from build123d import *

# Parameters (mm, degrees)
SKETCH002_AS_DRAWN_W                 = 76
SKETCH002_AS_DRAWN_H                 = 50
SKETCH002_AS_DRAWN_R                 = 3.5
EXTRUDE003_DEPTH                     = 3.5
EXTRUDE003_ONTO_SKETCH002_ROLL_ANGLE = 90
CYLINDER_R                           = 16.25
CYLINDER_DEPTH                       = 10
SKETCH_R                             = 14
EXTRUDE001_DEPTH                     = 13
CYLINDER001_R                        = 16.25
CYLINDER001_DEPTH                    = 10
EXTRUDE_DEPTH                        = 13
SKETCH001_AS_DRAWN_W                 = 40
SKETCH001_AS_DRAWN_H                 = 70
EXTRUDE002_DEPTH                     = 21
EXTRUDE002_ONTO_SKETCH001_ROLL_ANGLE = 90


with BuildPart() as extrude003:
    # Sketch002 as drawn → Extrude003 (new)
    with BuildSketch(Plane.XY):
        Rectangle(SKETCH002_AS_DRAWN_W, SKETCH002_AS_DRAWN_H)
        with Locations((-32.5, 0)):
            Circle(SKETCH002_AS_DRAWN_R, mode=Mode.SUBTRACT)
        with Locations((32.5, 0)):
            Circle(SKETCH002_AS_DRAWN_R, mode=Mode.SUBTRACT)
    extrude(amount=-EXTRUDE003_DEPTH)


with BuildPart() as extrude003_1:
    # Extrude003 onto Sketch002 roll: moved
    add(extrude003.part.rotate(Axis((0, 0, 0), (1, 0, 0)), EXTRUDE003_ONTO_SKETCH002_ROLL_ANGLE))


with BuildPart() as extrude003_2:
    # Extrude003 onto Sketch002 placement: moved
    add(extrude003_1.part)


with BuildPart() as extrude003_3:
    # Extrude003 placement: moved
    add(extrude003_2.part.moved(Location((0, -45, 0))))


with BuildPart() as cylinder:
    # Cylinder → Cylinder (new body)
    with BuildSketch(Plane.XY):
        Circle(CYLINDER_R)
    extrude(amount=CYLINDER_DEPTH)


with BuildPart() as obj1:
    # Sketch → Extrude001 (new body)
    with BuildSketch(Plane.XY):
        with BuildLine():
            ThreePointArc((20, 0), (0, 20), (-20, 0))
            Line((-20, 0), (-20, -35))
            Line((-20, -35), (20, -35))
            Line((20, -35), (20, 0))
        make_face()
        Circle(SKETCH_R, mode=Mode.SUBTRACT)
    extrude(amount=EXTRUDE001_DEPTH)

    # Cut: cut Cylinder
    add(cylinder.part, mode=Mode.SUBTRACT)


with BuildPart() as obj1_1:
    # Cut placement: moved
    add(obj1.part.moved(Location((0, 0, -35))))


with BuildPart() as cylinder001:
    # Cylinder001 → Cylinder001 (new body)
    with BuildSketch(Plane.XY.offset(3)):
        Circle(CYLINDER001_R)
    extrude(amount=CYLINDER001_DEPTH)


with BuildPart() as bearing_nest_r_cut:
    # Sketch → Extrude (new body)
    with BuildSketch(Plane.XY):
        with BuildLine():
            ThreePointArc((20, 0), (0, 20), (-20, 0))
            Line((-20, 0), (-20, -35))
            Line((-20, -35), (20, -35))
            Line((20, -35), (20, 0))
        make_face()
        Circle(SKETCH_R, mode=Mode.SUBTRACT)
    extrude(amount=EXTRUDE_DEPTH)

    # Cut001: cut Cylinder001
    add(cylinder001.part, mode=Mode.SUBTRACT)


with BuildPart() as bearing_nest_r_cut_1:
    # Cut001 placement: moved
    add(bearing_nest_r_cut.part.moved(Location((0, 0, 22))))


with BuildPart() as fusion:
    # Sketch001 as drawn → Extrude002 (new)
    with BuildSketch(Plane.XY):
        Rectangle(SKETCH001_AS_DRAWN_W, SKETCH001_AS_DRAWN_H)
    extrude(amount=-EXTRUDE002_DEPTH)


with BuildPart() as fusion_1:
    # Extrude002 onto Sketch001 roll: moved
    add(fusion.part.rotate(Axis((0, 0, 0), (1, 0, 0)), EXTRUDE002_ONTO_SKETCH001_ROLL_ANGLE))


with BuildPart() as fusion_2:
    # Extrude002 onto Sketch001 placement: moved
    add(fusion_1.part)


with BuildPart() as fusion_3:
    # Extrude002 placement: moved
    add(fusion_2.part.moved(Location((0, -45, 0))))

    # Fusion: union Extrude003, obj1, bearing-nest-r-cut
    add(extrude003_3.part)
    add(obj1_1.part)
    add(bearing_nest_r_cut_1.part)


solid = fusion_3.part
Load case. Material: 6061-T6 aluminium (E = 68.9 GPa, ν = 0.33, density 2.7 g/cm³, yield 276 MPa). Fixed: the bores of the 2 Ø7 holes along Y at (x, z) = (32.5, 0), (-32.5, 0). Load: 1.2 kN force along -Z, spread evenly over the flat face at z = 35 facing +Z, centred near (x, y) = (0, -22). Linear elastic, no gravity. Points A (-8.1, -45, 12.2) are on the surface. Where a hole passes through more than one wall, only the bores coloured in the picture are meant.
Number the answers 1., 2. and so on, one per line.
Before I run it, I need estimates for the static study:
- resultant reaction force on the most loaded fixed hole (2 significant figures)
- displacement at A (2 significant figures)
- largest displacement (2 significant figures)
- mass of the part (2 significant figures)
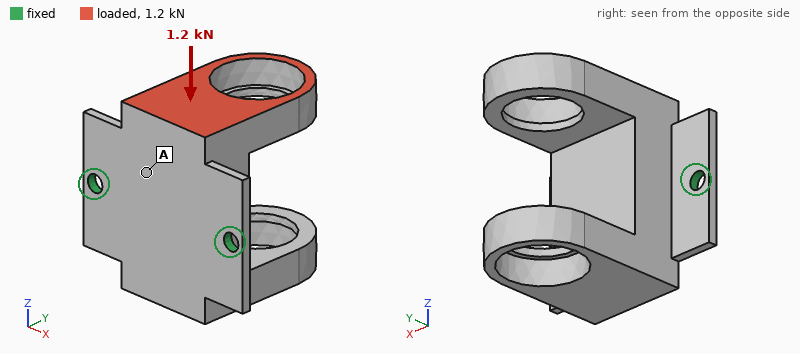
1. 600 N
2. 0.091 mm
3. 0.58 mm
4. 230 g
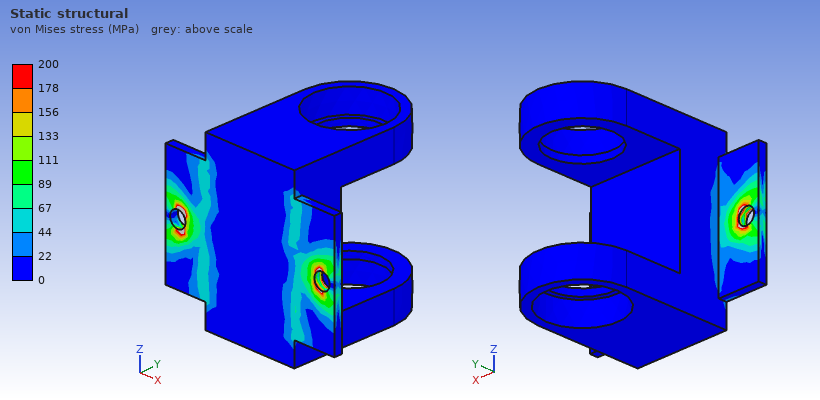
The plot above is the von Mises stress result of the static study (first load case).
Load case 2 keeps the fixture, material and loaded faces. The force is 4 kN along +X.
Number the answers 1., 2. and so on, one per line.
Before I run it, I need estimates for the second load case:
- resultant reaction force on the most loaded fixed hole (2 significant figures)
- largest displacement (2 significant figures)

1. 3.4 kN
2. 0.22 mm
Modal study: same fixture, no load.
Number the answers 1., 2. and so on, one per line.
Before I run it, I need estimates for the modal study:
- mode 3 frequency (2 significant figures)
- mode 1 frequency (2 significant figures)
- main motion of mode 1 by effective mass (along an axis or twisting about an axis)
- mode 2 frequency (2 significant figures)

1. 2600 Hz
2. 640 Hz
3. along Z
4. 2600 Hz
